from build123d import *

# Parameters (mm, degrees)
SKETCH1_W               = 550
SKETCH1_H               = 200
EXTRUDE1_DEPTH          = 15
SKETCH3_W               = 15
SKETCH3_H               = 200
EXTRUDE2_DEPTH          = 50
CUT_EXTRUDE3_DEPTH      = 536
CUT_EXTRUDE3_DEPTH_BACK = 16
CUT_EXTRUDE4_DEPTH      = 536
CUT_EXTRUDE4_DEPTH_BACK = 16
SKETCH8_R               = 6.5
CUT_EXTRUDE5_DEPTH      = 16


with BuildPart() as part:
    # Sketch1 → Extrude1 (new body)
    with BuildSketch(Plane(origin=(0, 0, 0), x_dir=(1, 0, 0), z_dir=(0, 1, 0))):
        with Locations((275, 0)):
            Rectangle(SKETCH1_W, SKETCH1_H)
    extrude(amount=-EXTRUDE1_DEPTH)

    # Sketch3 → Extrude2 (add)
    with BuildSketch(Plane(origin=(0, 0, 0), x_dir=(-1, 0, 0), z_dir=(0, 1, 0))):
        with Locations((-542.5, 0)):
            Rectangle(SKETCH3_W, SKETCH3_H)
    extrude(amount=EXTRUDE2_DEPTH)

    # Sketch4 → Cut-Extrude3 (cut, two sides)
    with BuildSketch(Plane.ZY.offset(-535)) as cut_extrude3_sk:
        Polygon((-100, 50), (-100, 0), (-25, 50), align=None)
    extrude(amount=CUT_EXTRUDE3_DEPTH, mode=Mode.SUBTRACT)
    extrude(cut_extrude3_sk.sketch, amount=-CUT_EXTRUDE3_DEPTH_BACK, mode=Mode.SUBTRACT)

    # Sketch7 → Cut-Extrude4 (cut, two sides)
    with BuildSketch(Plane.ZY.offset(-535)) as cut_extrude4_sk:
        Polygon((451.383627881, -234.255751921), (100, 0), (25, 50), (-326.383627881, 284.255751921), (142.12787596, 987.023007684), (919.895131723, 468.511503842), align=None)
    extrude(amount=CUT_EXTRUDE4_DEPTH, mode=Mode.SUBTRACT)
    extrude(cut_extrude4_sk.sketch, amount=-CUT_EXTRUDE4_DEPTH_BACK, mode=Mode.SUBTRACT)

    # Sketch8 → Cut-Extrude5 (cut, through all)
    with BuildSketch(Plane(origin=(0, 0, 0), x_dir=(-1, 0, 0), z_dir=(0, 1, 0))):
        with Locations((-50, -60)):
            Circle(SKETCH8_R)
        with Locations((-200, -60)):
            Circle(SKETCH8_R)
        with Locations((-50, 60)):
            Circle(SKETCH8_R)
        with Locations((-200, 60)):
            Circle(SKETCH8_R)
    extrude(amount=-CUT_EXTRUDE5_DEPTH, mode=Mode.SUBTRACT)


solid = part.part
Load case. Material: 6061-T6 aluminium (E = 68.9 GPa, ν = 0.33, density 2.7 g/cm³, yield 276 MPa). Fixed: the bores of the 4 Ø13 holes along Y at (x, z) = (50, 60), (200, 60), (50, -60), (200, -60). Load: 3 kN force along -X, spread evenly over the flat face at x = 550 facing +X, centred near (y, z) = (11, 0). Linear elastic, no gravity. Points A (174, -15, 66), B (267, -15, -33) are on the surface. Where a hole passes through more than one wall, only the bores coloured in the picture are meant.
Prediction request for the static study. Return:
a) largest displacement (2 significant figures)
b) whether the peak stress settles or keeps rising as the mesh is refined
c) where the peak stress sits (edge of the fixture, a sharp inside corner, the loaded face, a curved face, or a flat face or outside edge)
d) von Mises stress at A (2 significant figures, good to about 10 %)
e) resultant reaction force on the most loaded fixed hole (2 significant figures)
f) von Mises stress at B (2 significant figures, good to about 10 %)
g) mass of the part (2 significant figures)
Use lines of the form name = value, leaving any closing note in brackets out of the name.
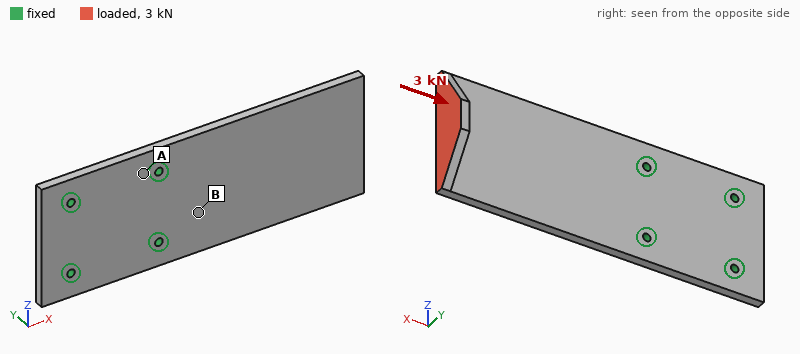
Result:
largest displacement = 0.93 mm
whether the peak stress settles or keeps rising as the mesh is refined = keeps rising
where the peak stress sits = edge of the fixture
von Mises stress at A = 1.8 MPa
resultant reaction force on the most loaded fixed hole = 1.3 kN
von Mises stress at B = 5.9 MPa
mass of the part = 4.7 kg
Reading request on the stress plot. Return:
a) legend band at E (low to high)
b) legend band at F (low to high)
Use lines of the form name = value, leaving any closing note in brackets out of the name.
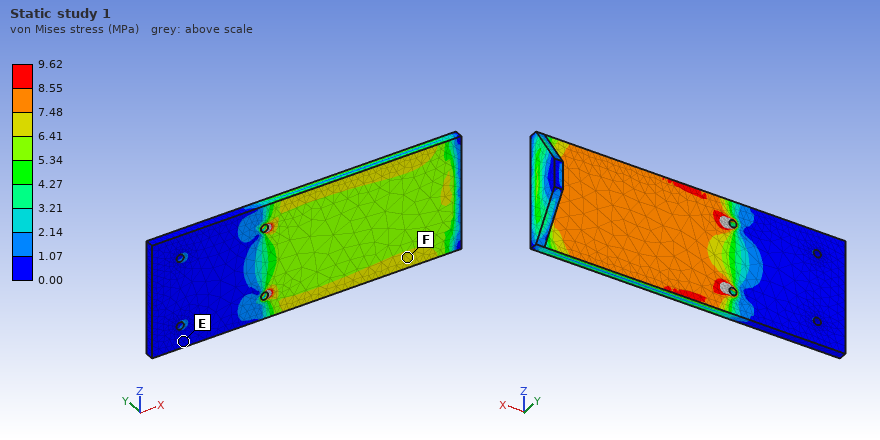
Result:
legend band at E = 0.00 to 1.07 MPa
legend band at F = 6.41 to 7.48 MPa
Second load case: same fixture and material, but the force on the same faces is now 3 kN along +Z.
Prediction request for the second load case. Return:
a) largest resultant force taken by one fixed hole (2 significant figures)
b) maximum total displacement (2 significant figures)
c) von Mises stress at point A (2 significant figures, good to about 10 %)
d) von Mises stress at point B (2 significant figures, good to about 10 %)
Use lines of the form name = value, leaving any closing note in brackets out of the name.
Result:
largest resultant force taken by one fixed hole = 6.8 kN
maximum total displacement = 0.30 mm
von Mises stress at point A = 2.8 MPa
von Mises stress at point B = 4.7 MPa
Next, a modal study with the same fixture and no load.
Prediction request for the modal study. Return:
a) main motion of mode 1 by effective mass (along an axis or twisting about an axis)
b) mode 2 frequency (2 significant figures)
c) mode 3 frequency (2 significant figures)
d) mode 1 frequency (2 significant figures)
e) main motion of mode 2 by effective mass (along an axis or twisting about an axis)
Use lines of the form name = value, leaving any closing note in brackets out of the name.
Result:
main motion of mode 1 by effective mass = along Y
mode 2 frequency = 350 Hz
mode 3 frequency = 540 Hz
mode 1 frequency = 85 Hz
main motion of mode 2 by effective mass = twisting about X
